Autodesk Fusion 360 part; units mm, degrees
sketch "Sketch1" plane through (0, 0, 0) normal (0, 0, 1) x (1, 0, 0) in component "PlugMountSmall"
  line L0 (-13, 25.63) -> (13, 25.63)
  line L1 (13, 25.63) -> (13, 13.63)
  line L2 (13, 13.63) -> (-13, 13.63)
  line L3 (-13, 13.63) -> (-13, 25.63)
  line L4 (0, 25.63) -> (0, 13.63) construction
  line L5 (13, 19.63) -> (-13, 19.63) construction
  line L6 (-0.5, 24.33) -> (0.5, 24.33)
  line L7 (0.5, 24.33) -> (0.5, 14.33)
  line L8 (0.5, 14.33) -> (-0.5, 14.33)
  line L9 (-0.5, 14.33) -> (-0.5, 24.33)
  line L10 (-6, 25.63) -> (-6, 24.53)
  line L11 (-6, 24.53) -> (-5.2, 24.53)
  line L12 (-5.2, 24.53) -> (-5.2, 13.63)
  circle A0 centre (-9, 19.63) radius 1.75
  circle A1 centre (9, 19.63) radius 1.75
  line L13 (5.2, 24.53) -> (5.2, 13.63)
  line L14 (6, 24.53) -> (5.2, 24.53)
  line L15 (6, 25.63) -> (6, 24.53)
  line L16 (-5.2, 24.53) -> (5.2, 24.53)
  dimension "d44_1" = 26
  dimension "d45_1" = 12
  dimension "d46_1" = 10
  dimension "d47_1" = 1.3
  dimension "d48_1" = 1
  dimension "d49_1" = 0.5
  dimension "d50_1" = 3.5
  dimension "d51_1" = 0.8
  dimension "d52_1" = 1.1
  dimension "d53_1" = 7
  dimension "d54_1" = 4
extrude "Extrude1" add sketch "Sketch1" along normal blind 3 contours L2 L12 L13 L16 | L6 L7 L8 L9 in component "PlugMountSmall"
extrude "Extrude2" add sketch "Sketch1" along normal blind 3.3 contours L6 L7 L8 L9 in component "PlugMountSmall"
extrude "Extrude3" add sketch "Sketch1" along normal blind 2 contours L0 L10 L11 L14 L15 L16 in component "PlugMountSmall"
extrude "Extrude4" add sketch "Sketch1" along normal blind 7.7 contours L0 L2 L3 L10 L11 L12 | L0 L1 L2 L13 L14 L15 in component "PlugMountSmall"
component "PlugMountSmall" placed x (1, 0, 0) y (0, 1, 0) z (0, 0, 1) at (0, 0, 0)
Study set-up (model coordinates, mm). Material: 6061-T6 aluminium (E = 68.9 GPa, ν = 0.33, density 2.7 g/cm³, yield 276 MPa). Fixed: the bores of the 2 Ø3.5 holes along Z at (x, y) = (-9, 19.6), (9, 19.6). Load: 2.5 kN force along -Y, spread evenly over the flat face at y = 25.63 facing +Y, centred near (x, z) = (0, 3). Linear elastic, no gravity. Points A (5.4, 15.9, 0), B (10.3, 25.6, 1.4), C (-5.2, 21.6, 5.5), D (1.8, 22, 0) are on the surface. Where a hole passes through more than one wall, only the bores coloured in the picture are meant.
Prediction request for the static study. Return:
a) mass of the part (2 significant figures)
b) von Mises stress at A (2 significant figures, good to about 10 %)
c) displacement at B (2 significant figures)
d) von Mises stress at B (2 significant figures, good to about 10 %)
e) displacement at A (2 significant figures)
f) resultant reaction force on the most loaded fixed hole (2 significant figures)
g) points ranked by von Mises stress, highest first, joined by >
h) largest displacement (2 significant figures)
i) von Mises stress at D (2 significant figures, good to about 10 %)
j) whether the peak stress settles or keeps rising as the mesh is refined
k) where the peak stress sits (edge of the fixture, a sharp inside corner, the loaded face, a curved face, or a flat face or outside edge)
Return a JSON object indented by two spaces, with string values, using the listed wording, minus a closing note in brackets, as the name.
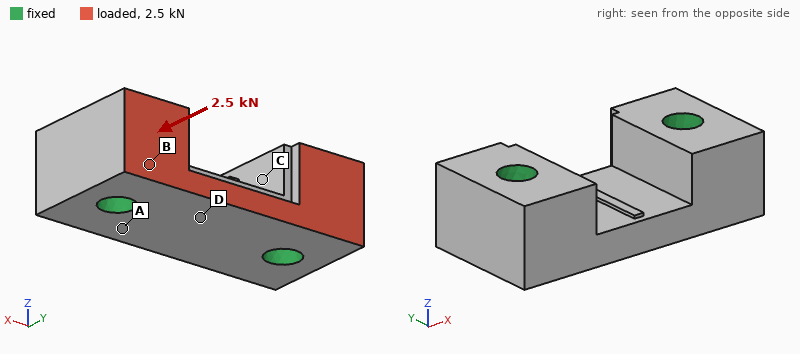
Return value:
{
  "mass of the part": "4.5 g",
  "von Mises stress at A": "9.7 MPa",
  "displacement at B": "1.6 µm",
  "von Mises stress at B": "22 MPa",
  "displacement at A": "0.92 µm",
  "resultant reaction force on the most loaded fixed hole": "1.3 kN",
  "points ranked by von Mises stress, highest first, joined by >": "B > D > A > C",
  "largest displacement": "4.0 µm",
  "von Mises stress at D": "16 MPa",
  "whether the peak stress settles or keeps rising as the mesh is refined": "keeps rising",
  "where the peak stress sits": "edge of the fixture"
}
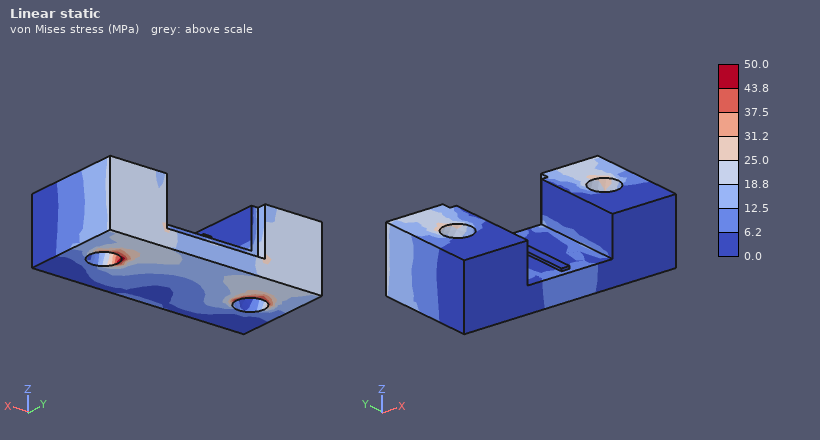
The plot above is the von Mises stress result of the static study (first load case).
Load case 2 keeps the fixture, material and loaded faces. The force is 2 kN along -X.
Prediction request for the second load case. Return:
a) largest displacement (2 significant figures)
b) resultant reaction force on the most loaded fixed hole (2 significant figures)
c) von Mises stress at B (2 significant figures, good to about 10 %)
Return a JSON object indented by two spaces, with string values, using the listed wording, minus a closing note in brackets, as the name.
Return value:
{
  "largest displacement": "7.6 µm",
  "resultant reaction force on the most loaded fixed hole": "1.0 kN",
  "von Mises stress at B": "35 MPa"
}
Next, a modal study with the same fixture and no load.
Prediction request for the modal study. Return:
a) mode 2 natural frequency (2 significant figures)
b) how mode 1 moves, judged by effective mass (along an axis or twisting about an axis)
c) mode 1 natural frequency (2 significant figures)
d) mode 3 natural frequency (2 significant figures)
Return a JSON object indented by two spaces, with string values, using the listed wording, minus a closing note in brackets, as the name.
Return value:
{
  "mode 2 natural frequency": "69 kHz",
  "how mode 1 moves, judged by effective mass": "along Z",
  "mode 1 natural frequency": "65 kHz",
  "mode 3 natural frequency": "77 kHz"
}
